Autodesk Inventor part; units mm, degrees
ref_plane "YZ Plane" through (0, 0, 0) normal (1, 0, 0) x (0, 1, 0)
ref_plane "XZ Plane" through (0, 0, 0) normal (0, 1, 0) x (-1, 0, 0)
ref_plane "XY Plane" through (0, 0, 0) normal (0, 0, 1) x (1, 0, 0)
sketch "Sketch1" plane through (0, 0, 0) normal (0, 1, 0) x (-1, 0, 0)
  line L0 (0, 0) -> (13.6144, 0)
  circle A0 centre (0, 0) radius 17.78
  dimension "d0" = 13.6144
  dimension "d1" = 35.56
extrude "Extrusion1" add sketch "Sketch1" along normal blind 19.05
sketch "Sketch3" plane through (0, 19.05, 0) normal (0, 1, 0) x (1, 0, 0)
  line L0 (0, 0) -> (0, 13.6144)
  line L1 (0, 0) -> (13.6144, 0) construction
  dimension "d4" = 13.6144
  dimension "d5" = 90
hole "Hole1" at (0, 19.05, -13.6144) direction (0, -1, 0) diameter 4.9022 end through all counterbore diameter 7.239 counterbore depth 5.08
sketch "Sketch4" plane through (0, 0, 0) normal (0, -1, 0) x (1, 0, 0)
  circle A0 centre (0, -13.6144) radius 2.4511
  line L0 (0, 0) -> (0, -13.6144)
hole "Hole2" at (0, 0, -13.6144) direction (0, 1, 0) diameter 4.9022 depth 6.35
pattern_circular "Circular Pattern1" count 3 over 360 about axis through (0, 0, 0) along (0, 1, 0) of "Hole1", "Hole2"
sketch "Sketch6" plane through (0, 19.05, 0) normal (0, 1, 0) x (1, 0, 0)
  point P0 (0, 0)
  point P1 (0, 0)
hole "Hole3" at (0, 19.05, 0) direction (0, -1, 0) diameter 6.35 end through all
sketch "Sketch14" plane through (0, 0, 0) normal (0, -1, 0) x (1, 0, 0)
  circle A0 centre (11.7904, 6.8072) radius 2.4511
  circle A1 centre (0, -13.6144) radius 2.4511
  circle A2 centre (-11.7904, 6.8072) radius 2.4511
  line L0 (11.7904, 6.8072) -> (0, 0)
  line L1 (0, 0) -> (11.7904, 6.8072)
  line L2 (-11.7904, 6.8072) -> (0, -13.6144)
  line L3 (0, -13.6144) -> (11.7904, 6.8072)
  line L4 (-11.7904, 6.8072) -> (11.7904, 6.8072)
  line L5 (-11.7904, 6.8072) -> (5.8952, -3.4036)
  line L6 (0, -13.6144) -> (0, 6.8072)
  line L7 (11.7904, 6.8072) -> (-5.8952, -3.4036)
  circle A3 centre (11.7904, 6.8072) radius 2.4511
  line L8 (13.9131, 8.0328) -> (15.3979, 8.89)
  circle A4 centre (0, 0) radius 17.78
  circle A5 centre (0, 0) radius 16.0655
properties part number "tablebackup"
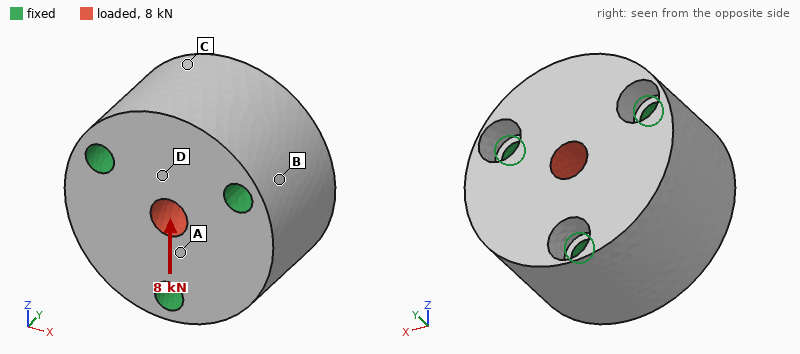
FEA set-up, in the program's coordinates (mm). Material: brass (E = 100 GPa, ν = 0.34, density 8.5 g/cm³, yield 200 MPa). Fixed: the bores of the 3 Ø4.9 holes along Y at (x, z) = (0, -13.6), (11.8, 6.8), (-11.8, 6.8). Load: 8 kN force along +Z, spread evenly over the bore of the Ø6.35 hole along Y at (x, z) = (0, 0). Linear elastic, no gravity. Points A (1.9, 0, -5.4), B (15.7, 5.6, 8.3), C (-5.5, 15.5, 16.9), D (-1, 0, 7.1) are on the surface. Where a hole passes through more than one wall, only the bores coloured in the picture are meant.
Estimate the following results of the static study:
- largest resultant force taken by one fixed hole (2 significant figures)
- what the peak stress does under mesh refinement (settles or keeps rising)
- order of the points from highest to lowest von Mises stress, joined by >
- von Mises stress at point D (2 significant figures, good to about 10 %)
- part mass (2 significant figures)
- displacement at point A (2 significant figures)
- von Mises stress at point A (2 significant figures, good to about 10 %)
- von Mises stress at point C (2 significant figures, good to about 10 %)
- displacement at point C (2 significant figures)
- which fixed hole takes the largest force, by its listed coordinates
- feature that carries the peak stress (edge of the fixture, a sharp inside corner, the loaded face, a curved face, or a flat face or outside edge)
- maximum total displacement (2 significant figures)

3.0 kN
keeps rising
A > D > C > B
13 MPa
140 g
1.3 µm
21 MPa
8.0 MPa
2.0 µm
(0, -13.6)
edge of the fixture
3.6 µm
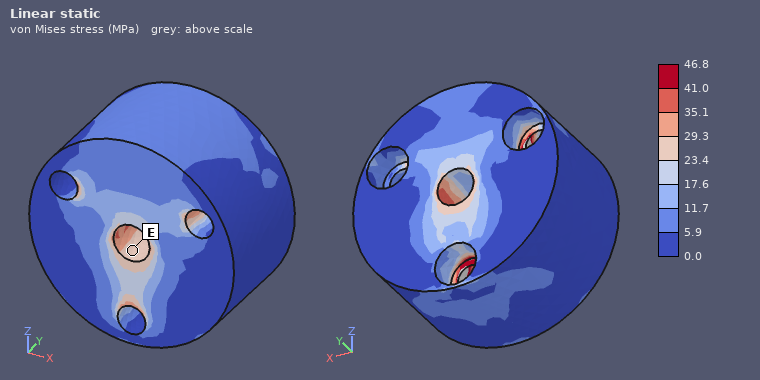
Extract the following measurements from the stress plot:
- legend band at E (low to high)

23.4 to 29.3 MPa
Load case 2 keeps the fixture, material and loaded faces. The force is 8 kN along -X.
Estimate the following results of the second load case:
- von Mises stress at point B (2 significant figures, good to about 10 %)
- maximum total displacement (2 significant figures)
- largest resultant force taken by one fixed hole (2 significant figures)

4.8 MPa
3.4 µm
2.9 kN
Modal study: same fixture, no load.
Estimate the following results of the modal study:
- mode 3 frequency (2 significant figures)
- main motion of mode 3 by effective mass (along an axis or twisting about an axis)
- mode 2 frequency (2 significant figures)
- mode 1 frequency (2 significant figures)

32 kHz
along Y
27 kHz
27 kHz
